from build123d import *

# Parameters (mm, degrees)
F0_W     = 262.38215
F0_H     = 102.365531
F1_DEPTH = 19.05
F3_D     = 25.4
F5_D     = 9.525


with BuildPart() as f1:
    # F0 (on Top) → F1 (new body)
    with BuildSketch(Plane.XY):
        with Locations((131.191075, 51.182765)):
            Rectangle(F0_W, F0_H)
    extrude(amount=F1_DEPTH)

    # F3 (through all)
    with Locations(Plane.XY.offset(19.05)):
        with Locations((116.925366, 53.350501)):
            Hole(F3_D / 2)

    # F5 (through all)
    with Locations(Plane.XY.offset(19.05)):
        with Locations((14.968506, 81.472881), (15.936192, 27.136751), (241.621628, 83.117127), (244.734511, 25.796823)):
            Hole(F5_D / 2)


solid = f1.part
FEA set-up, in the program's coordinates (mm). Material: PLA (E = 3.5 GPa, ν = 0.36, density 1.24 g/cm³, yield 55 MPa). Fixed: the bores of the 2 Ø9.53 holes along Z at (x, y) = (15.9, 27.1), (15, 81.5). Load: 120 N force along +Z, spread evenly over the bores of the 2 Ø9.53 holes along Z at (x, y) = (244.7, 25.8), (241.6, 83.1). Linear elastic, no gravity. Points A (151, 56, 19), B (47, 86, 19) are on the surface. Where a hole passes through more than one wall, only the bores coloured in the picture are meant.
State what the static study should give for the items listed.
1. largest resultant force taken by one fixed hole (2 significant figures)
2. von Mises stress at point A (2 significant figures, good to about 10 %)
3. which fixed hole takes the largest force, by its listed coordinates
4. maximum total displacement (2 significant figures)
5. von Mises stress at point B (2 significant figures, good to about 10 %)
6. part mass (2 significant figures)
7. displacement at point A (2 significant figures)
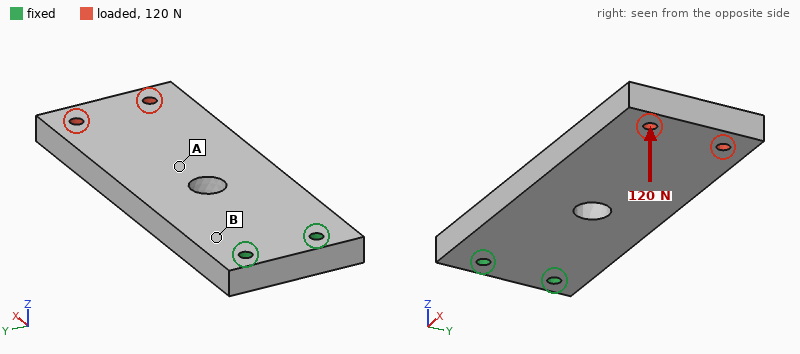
71 N
1.5 MPa
(15.9, 27.1)
2.8 mm
3.8 MPa
620 g
1.1 mm
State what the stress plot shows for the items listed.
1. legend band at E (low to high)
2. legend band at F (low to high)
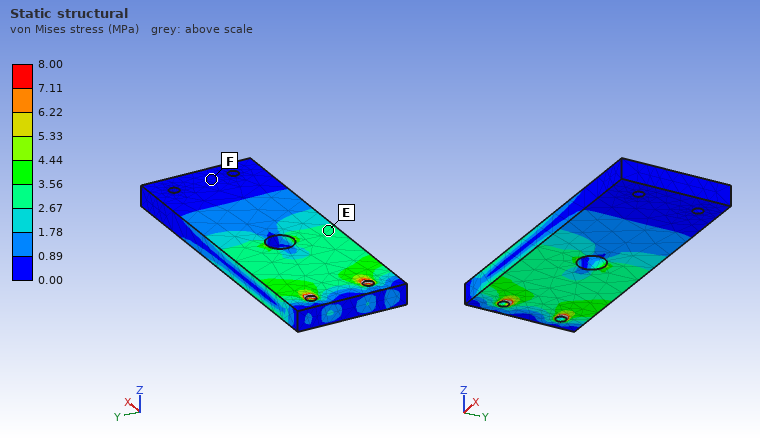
2.67 to 3.56 MPa
0.00 to 0.89 MPa
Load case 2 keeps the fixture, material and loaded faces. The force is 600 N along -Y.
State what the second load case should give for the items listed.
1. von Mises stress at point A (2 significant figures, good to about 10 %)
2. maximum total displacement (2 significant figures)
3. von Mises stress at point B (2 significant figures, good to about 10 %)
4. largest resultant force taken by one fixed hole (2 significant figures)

1.0 MPa
0.66 mm
2.8 MPa
2.3 kN
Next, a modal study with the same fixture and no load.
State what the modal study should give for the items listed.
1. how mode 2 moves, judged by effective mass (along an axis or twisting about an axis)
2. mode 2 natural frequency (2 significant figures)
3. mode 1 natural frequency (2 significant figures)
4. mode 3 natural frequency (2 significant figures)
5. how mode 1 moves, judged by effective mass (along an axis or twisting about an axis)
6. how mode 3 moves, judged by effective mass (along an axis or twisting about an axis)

along Y
350 Hz
82 Hz
380 Hz
along Z
twisting about X
